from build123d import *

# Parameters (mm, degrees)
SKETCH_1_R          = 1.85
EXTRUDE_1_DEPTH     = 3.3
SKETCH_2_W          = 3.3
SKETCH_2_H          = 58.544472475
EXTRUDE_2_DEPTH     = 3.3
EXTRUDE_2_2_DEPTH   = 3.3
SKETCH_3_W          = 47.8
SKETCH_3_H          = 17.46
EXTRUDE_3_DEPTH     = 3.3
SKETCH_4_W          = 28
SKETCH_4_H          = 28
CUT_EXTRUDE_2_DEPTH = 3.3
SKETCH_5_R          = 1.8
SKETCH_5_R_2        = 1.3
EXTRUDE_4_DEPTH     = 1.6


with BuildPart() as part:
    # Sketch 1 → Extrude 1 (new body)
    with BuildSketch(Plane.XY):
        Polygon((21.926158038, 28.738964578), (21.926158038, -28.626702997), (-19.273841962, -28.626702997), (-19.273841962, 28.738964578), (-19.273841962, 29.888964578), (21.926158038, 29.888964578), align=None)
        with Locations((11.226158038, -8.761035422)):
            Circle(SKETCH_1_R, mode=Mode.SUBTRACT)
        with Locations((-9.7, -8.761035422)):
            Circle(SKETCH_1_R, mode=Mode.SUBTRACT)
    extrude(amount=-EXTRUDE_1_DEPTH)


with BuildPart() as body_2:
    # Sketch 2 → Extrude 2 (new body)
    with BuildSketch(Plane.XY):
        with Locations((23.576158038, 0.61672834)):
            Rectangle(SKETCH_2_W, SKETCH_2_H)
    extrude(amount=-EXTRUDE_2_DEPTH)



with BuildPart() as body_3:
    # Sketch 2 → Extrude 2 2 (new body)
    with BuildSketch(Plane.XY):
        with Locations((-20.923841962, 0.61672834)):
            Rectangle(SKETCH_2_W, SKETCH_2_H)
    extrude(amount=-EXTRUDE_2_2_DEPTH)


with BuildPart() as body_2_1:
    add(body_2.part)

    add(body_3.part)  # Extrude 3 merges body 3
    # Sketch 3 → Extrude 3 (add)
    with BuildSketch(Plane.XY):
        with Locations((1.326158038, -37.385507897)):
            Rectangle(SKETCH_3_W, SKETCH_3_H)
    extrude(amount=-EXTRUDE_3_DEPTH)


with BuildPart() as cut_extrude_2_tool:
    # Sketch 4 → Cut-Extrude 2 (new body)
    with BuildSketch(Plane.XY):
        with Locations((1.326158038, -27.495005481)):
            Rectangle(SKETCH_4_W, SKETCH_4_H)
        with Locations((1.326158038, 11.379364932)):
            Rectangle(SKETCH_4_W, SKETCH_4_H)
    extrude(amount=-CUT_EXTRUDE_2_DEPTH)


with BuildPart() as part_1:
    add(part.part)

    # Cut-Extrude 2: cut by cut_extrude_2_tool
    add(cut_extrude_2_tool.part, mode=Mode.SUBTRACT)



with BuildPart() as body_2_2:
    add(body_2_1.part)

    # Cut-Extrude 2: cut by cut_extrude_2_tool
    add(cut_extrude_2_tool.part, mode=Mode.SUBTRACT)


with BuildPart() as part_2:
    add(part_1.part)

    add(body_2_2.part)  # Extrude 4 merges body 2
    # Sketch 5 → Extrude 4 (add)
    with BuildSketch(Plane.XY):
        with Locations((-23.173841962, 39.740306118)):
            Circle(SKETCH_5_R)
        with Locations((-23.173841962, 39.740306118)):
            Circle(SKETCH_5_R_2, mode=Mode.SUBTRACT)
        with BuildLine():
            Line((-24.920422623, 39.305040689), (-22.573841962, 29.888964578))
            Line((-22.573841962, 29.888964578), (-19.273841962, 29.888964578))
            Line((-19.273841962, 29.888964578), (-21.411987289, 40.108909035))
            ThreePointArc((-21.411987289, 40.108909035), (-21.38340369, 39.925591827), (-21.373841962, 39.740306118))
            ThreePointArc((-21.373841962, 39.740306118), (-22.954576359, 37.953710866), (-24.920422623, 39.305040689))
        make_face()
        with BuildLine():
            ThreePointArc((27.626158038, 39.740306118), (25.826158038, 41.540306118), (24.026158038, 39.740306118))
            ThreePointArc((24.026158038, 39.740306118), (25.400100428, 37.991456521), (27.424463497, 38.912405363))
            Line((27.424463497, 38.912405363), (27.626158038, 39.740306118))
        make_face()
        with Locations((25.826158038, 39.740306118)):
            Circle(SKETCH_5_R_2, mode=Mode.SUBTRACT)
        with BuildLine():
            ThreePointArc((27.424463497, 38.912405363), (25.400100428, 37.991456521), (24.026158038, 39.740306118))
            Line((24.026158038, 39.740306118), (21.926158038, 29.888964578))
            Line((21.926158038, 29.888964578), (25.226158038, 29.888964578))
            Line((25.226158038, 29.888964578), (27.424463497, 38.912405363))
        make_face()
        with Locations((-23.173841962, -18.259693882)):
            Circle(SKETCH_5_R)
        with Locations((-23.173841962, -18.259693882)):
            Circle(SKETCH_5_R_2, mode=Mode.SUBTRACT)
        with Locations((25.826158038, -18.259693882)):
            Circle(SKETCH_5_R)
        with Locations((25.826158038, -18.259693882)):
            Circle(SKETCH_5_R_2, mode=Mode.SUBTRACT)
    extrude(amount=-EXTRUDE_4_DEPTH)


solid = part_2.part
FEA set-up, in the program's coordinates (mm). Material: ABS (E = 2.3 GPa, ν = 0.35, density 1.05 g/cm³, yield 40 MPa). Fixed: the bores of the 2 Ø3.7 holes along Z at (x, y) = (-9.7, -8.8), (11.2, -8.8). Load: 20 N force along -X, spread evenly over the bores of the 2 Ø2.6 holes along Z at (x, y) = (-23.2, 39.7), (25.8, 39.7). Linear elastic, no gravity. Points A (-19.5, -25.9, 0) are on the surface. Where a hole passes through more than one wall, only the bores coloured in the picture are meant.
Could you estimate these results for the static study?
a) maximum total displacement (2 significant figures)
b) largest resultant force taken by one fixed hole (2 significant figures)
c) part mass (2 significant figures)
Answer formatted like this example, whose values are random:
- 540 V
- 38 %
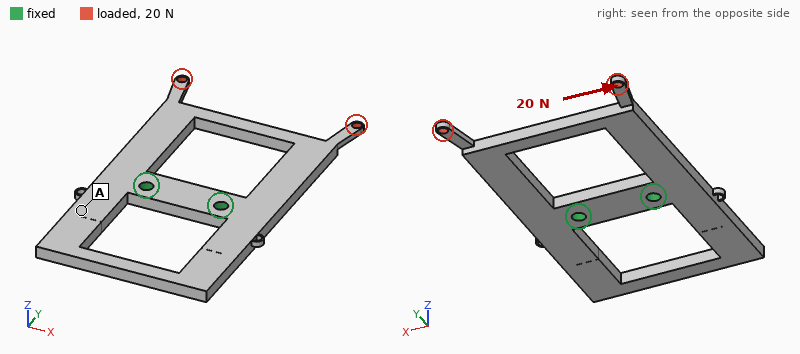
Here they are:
- 1.2 mm
- 27 N
- 7.2 g
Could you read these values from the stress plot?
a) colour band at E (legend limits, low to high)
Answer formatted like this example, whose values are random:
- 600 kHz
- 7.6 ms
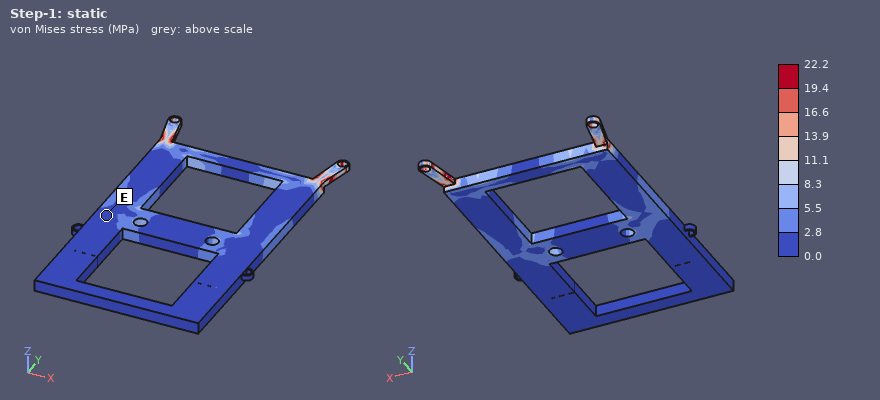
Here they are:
- 0.0 to 2.8 MPa
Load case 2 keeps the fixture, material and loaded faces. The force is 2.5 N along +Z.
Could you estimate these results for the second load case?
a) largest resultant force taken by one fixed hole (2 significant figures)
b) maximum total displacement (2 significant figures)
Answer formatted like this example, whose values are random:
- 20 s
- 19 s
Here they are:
- 1.3 N
- 1.1 mm
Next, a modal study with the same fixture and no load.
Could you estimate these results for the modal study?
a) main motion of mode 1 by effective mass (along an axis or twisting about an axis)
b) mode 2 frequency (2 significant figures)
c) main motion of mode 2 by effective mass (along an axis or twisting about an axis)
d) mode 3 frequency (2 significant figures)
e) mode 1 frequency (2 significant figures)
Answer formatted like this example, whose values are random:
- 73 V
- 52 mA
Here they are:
- twisting about X
- 420 Hz
- along Z
- 620 Hz
- 350 Hz
